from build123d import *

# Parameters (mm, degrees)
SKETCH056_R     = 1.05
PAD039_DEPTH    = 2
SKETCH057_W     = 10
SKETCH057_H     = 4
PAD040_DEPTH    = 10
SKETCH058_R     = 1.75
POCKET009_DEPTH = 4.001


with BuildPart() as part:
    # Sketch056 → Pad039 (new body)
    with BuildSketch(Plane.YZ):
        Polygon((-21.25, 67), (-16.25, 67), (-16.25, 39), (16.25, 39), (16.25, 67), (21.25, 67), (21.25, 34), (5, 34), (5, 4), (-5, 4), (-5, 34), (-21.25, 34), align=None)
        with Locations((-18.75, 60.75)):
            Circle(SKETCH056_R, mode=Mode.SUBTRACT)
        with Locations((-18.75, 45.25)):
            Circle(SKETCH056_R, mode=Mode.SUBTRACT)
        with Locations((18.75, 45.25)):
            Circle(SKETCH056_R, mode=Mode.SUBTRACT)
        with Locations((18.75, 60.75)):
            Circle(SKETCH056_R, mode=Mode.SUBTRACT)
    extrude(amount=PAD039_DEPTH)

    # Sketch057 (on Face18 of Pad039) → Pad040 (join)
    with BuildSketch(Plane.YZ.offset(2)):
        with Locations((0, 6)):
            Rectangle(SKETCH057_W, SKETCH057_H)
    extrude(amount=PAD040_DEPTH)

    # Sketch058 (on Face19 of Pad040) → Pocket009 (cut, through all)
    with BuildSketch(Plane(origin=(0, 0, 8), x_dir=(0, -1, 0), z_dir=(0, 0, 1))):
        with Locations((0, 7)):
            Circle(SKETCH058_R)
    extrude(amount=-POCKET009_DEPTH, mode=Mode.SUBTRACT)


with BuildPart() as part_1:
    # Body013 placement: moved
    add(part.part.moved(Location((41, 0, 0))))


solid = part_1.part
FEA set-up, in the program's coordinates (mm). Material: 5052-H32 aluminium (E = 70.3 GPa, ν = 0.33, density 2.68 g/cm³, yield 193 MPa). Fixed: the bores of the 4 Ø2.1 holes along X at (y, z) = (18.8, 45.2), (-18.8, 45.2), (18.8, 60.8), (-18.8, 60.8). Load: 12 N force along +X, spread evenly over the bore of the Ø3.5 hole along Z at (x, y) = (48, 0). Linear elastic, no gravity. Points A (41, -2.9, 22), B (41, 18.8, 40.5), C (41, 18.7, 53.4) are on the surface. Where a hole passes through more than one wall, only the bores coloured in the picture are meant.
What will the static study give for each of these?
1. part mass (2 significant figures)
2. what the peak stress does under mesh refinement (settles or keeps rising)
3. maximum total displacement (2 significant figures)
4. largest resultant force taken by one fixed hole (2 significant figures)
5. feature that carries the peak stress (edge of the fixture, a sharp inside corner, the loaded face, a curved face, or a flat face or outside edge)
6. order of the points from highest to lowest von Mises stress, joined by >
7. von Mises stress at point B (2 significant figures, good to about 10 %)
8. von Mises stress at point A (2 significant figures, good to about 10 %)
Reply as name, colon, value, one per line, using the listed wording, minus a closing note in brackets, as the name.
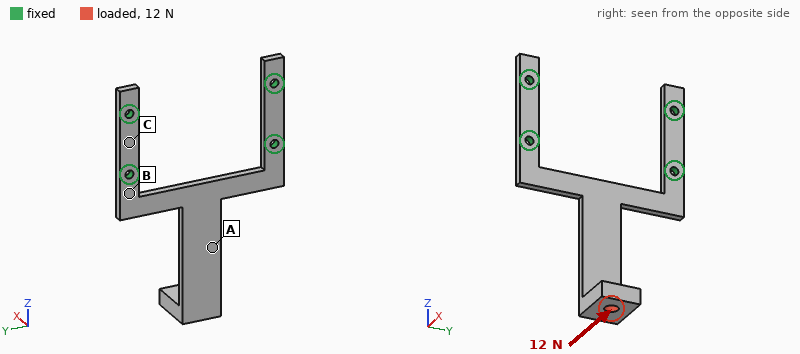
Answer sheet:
part mass: 5.1 g
what the peak stress does under mesh refinement: keeps rising
maximum total displacement: 0.88 mm
largest resultant force taken by one fixed hole: 6.2 N
feature that carries the peak stress: edge of the fixture
order of the points from highest to lowest von Mises stress, joined by >: B > A > C
von Mises stress at point B: 62 MPa
von Mises stress at point A: 29 MPa
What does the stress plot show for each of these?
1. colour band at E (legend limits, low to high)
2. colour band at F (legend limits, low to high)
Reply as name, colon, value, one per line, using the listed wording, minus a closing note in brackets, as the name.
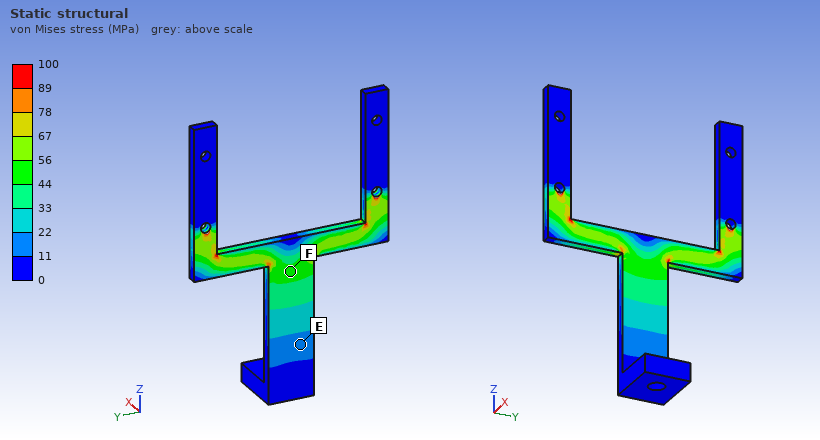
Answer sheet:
colour band at E: 11 to 22 MPa
colour band at F: 44 to 56 MPa
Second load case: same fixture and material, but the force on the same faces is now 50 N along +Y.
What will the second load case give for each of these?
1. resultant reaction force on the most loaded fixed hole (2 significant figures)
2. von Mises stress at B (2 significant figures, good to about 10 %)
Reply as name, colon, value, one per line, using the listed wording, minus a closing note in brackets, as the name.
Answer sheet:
resultant reaction force on the most loaded fixed hole: 58 N
von Mises stress at B: 20 MPa
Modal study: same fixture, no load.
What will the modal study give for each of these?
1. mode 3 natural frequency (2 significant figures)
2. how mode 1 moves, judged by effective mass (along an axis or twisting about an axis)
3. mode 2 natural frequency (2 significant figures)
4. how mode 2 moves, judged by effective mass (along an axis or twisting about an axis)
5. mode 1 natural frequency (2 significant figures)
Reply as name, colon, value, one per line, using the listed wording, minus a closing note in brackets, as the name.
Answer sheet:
mode 3 natural frequency: 3100 Hz
how mode 1 moves, judged by effective mass: along X
mode 2 natural frequency: 2300 Hz
how mode 2 moves, judged by effective mass: along Y
mode 1 natural frequency: 490 Hz
